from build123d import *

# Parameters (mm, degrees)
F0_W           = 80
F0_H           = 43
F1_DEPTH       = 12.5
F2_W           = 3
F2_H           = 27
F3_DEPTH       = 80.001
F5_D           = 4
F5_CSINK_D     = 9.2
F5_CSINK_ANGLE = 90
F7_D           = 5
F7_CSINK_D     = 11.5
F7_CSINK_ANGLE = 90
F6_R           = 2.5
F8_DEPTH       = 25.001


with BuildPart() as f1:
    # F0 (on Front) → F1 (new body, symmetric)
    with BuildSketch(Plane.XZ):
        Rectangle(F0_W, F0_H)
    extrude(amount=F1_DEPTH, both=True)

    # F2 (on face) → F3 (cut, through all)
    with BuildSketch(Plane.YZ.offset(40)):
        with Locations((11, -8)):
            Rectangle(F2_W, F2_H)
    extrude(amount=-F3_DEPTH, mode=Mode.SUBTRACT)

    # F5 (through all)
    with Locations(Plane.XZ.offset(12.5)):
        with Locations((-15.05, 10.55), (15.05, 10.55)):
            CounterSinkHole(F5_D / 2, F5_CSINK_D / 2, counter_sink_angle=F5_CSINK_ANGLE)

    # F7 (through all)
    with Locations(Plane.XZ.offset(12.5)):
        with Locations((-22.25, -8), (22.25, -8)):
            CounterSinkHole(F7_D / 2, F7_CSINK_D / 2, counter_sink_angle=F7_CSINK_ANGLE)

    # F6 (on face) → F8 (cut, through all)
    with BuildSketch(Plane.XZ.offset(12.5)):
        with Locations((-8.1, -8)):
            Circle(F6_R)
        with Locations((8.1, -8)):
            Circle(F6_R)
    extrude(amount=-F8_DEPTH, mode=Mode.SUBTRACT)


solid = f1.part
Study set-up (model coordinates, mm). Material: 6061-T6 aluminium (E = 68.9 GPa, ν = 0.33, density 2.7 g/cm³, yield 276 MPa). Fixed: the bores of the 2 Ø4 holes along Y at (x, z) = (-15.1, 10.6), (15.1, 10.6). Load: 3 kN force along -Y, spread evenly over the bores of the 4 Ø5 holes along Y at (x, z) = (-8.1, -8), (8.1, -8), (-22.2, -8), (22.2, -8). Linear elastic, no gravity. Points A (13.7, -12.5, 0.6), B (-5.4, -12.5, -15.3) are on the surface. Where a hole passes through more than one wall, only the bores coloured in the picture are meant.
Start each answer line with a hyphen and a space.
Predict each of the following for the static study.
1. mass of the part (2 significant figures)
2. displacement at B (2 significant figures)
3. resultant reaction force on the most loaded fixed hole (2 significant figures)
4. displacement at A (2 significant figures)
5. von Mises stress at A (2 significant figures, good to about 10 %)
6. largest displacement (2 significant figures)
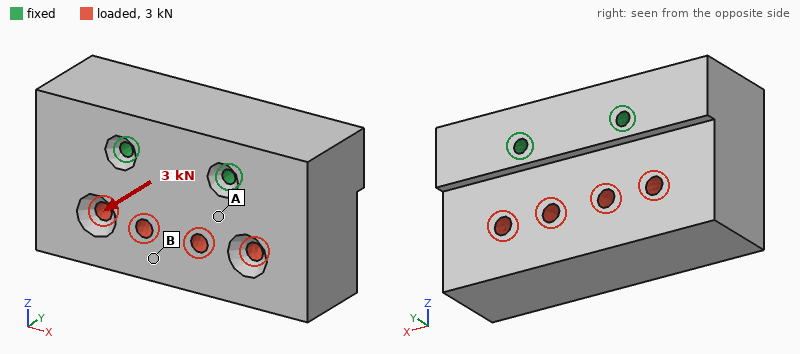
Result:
- 210 g
- 8.1 µm
- 1.5 kN
- 4.0 µm
- 5.1 MPa
- 9.5 µm
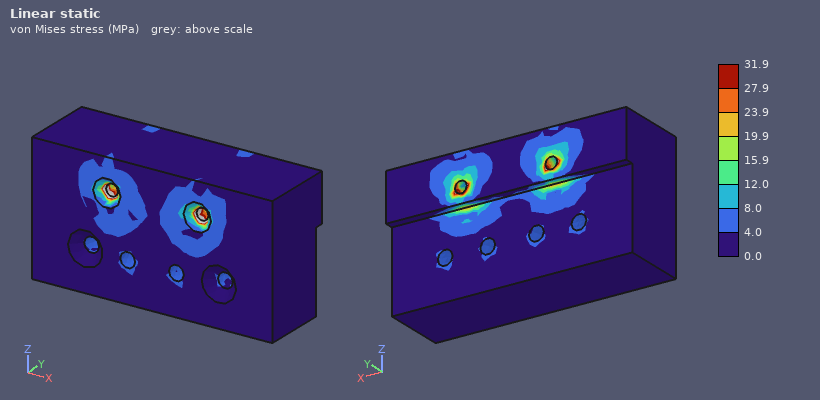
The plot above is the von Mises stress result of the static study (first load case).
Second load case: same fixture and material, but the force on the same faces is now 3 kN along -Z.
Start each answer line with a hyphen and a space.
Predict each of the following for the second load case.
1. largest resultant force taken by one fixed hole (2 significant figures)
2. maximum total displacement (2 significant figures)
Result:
- 1.5 kN
- 1.2 µm
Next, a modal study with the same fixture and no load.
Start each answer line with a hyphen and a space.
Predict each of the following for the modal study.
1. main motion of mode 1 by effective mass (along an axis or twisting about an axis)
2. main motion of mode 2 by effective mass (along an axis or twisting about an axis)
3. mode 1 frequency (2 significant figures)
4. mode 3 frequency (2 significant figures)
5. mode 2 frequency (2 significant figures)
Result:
- along Y
- along X
- 9200 Hz
- 11 kHz
- 10 kHz
